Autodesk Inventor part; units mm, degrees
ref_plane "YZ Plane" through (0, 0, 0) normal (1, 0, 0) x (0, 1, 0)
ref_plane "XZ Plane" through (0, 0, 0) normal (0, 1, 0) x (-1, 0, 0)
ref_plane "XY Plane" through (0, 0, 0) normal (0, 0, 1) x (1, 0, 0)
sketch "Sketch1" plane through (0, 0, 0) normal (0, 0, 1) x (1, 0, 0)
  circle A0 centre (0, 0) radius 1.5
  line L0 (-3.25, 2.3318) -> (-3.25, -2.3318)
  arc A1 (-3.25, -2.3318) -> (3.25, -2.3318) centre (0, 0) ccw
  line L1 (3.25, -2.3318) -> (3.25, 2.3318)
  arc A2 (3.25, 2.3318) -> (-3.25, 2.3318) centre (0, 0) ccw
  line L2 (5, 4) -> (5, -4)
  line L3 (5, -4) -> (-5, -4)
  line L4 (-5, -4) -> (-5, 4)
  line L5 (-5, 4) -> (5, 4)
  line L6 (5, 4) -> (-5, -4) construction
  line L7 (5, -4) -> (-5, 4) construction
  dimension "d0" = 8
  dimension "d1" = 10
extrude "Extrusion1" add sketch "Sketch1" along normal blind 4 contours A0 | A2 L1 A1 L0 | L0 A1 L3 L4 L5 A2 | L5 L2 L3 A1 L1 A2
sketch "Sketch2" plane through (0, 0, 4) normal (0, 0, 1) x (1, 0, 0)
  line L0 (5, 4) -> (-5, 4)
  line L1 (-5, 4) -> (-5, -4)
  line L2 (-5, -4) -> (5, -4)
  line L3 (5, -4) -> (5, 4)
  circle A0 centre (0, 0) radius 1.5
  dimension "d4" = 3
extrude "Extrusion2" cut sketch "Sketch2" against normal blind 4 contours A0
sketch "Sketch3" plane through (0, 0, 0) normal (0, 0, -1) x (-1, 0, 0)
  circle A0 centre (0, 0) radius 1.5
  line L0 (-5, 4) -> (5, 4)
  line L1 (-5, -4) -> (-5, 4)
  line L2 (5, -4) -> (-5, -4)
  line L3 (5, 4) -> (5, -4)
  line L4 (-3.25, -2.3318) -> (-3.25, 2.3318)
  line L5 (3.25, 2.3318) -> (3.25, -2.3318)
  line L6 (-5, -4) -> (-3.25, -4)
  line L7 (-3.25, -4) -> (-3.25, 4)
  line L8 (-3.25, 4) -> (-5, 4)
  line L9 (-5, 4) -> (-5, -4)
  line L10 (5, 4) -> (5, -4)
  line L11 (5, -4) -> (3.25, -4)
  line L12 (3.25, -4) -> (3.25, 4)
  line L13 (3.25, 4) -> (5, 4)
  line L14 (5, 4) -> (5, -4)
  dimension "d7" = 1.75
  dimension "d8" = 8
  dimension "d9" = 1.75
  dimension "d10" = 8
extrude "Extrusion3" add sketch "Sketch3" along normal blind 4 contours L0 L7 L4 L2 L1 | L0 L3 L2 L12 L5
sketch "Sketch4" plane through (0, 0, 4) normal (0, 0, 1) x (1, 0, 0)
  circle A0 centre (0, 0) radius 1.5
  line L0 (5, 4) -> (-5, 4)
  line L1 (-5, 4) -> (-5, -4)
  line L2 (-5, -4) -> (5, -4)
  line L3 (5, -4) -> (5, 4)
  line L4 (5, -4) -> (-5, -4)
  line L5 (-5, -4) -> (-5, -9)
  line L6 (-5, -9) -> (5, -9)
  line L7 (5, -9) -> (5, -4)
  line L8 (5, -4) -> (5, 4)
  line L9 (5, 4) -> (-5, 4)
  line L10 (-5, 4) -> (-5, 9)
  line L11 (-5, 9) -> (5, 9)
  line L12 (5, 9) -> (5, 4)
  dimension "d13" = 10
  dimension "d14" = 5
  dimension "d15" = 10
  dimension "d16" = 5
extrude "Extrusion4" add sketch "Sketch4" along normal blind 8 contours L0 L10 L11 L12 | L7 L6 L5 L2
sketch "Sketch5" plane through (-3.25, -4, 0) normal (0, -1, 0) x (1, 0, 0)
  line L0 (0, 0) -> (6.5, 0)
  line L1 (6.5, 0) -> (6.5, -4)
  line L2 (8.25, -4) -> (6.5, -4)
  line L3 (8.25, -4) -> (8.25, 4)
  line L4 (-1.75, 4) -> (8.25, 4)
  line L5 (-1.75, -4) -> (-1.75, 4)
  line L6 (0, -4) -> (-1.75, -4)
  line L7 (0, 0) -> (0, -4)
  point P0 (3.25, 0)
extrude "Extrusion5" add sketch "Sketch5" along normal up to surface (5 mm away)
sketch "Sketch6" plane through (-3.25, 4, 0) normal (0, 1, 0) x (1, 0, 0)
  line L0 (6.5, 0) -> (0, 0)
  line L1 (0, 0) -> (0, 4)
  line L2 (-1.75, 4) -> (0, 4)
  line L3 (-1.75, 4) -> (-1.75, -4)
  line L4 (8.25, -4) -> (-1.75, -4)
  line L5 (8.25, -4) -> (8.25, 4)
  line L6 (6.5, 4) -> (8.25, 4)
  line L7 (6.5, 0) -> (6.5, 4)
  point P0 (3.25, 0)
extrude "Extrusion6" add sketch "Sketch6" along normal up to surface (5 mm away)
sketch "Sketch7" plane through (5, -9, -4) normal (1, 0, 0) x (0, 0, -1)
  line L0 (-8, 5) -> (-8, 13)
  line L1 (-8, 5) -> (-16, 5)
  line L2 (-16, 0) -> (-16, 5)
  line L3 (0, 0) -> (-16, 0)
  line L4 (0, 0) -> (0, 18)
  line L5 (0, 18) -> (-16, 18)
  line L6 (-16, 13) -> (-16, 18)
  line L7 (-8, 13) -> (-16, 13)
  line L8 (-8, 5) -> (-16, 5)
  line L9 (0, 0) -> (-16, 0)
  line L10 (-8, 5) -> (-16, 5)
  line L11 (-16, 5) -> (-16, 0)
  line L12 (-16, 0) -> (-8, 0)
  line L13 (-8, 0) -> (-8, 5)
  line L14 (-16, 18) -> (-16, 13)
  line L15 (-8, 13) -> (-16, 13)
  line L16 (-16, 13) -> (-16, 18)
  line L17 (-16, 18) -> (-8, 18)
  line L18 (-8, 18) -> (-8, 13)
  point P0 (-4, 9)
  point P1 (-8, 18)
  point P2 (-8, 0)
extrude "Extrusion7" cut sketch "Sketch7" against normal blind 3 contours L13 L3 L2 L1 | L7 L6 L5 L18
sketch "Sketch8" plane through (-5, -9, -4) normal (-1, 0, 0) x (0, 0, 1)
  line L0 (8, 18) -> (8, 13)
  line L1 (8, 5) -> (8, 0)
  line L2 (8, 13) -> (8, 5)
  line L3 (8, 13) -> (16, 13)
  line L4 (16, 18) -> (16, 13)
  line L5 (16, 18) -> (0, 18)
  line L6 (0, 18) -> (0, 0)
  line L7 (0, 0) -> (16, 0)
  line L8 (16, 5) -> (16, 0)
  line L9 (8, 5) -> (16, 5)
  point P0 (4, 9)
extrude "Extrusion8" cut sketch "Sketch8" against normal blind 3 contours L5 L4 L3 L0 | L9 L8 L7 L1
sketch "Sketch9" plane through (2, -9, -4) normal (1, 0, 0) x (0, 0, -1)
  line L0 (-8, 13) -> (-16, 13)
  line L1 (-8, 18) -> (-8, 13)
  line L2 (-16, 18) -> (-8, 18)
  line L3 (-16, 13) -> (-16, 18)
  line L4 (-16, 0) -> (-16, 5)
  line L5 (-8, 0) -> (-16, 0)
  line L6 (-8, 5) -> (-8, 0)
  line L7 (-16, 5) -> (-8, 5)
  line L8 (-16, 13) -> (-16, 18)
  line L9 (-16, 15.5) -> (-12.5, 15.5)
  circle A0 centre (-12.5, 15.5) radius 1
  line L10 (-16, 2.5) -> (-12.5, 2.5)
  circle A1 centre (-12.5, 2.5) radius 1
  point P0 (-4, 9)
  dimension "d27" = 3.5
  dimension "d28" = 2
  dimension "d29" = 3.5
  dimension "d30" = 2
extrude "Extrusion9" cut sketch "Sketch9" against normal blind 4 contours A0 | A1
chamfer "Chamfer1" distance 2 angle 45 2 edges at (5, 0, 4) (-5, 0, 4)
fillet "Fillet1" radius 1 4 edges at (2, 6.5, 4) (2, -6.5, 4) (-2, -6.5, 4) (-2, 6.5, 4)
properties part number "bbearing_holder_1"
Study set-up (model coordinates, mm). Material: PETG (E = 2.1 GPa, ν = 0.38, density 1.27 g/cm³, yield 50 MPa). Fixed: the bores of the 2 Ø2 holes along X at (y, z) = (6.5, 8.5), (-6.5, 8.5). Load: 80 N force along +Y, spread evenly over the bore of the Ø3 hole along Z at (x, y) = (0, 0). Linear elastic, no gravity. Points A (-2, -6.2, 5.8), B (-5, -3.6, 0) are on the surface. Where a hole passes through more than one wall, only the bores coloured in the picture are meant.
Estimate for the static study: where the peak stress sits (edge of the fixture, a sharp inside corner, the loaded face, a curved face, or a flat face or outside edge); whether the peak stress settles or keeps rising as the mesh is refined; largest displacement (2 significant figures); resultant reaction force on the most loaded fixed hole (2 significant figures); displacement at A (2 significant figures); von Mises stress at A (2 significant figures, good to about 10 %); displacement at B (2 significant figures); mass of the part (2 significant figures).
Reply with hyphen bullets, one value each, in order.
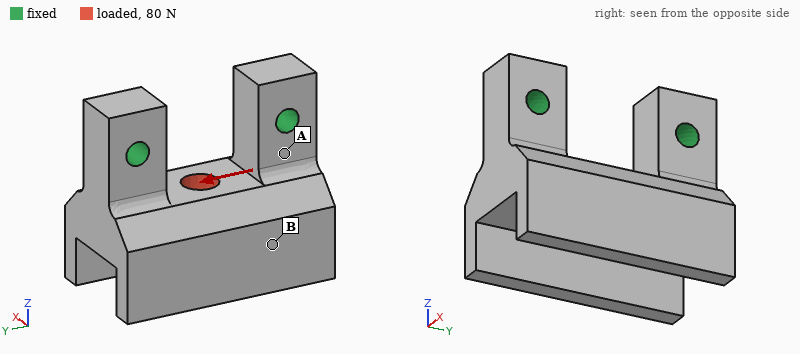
- edge of the fixture
- keeps rising
- 34 µm
- 46 N
- 12 µm
- 5.7 MPa
- 31 µm
- 1.5 g
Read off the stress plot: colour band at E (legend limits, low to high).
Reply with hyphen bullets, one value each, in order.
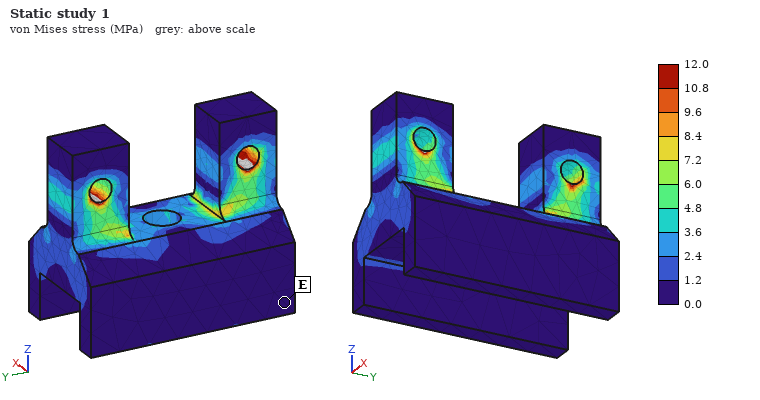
- 0.0 to 1.2 MPa
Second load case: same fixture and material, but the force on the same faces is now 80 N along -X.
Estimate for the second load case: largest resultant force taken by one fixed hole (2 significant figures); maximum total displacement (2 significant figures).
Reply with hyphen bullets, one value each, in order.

- 40 N
- 0.18 mm
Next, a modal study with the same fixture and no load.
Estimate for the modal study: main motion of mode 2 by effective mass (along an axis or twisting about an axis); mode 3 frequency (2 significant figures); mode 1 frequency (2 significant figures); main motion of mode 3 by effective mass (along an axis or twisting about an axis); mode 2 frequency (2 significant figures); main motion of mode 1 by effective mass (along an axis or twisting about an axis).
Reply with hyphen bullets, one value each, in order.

- twisting about Z
- 7300 Hz
- 3400 Hz
- along Y
- 6700 Hz
- along X
